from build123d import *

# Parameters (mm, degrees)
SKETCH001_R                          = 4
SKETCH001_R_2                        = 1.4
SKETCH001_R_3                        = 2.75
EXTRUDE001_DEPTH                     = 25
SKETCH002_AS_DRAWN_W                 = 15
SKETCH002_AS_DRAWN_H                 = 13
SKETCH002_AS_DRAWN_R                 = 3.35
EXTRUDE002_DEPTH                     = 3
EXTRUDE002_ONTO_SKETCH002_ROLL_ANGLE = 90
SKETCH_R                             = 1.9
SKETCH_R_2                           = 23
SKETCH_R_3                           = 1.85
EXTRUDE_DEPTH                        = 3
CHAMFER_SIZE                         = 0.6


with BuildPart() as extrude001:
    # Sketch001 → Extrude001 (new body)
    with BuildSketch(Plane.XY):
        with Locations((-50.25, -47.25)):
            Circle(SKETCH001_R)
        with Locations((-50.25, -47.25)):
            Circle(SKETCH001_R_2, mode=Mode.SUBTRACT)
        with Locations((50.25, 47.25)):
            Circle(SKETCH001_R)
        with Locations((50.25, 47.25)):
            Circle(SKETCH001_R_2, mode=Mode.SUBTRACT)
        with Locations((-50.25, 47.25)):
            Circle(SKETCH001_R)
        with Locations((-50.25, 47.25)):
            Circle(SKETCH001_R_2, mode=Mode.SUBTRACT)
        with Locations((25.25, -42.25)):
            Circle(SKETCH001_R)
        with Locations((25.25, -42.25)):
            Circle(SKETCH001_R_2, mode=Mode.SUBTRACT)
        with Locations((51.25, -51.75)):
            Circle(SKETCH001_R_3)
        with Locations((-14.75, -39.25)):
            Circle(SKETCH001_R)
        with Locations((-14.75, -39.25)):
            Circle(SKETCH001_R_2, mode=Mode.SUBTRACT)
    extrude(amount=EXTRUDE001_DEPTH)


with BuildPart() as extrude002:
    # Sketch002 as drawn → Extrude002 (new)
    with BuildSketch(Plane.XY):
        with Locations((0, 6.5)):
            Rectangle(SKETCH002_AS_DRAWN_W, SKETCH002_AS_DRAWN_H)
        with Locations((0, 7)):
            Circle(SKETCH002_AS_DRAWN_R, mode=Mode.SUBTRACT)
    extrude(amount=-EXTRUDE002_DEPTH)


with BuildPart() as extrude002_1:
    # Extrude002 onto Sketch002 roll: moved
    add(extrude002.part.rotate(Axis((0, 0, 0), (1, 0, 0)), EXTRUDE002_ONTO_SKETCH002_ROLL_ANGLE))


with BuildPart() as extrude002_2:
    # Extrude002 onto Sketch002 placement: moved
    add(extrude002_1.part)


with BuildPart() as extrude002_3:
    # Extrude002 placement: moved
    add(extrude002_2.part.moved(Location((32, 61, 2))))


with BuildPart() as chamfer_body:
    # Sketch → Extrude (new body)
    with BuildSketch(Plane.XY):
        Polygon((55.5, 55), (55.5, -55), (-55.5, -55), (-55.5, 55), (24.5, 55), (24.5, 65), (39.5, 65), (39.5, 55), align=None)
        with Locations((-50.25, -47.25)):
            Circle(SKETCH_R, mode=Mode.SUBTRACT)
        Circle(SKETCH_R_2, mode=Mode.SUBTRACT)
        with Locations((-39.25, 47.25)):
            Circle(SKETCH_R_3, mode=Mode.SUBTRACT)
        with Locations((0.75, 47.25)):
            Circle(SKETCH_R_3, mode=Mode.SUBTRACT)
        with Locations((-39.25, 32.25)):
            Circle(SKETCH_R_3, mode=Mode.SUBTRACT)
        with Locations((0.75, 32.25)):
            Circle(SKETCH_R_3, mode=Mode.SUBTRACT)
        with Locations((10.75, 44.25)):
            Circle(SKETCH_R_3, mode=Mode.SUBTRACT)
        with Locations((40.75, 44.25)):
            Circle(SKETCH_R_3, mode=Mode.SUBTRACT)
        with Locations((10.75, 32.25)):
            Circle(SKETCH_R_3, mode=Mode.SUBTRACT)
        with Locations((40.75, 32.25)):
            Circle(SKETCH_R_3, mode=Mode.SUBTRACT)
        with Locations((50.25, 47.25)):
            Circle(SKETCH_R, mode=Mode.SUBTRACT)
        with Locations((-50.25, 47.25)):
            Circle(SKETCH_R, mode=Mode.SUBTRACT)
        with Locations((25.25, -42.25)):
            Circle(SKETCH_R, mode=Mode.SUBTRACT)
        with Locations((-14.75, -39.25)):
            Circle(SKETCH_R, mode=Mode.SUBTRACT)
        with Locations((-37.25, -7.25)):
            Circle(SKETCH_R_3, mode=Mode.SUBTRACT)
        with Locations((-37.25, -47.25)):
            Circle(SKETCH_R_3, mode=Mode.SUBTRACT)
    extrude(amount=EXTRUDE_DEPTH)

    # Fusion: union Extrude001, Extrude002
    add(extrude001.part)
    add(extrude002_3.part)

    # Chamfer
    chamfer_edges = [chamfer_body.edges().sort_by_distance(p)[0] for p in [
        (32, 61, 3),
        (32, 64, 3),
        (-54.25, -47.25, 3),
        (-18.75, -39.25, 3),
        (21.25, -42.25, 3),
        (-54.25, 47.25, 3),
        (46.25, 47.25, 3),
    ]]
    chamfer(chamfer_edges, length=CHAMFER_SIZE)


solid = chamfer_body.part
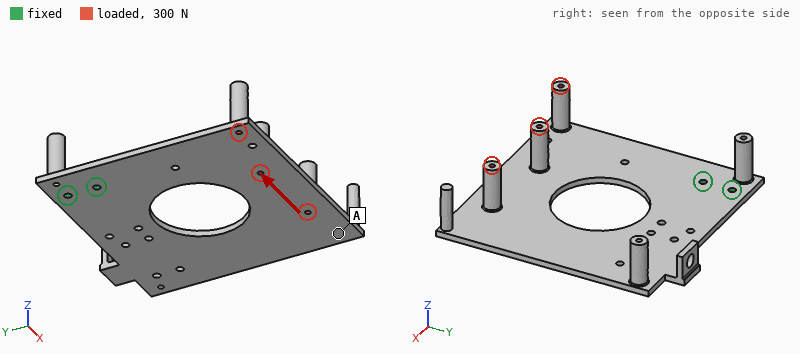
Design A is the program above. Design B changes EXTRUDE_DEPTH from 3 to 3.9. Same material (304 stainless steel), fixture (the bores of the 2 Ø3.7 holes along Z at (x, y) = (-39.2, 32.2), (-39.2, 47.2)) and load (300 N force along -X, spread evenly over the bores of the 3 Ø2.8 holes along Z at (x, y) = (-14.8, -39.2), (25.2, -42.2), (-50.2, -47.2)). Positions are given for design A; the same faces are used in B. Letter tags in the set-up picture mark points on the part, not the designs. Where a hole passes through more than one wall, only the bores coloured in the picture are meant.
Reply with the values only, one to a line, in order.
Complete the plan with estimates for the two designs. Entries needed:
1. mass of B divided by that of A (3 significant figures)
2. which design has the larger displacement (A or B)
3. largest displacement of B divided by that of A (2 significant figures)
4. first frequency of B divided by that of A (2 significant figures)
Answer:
1.25
A
0.45
1.3
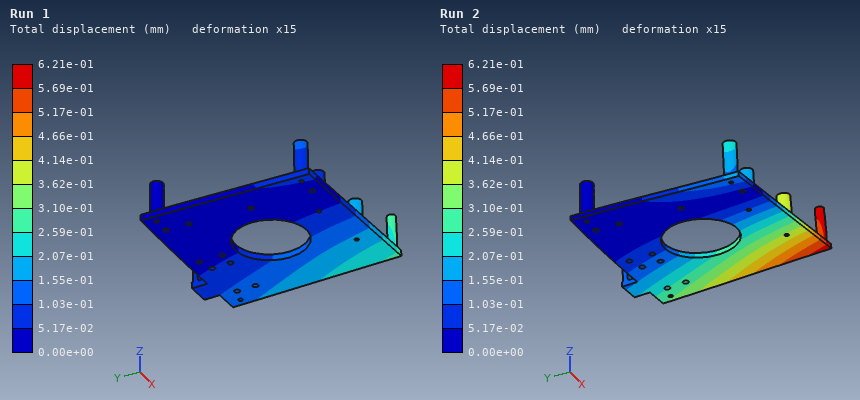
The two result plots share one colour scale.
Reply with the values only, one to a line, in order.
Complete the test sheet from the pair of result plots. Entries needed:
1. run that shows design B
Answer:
Run 1
